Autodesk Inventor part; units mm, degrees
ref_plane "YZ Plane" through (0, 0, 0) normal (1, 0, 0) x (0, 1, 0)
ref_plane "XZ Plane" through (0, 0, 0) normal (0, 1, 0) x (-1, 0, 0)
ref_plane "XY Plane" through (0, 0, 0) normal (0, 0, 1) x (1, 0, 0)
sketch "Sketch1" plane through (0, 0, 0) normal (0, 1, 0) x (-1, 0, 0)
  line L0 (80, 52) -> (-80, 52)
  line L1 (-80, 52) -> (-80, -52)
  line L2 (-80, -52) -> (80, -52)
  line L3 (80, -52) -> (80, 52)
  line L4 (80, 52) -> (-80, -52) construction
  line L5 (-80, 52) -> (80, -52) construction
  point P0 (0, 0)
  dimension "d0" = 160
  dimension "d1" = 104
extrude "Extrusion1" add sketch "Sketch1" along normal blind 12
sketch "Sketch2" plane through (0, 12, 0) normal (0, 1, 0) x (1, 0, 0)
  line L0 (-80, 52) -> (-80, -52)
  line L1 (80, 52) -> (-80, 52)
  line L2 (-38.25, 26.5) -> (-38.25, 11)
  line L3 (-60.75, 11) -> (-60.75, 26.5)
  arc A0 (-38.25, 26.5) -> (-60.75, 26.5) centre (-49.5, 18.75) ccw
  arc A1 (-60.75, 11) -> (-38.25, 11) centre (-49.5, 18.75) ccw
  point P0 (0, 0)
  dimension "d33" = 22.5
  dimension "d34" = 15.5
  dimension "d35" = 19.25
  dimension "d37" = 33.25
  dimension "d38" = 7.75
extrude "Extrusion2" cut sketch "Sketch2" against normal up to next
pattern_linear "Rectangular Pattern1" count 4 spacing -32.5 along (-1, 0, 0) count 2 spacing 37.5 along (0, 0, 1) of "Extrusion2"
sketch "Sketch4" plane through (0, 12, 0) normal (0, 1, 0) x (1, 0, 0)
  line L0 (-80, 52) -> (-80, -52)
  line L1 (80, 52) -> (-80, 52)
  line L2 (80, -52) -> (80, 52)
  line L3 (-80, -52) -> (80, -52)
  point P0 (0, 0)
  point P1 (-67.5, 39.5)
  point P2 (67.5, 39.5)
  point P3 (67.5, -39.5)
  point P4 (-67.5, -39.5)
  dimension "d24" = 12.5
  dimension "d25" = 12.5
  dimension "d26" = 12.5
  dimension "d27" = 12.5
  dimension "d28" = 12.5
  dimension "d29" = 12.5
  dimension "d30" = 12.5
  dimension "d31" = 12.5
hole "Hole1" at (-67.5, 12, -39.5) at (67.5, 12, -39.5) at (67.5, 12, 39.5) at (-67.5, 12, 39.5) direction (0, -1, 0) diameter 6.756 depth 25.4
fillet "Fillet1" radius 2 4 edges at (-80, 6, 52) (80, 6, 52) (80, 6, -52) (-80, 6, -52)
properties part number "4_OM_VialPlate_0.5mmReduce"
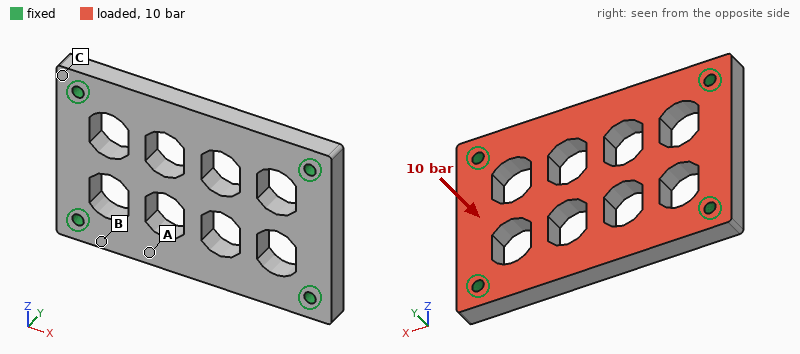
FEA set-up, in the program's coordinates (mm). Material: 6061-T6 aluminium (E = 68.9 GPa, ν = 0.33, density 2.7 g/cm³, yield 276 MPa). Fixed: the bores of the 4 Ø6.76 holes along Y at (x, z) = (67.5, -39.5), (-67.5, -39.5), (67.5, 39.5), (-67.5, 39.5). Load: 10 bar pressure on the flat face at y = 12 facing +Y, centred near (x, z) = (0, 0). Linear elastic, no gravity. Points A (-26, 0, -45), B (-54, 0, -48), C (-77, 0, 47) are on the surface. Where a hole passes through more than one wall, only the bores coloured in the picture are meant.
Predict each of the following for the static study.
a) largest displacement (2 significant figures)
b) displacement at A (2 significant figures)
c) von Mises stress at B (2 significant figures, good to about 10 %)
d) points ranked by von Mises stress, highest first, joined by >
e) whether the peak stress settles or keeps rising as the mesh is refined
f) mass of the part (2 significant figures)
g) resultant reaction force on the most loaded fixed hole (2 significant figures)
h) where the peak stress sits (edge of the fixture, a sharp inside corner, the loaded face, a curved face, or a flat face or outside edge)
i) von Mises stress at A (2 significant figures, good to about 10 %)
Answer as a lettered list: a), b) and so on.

a) 0.14 mm
b) 0.091 mm
c) 37 MPa
d) B > A > C
e) keeps rising
f) 400 g
g) 3.1 kN
h) edge of the fixture
i) 24 MPa
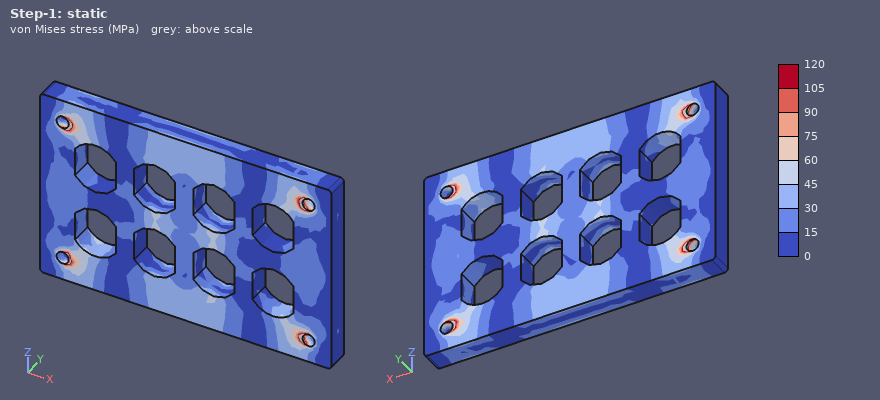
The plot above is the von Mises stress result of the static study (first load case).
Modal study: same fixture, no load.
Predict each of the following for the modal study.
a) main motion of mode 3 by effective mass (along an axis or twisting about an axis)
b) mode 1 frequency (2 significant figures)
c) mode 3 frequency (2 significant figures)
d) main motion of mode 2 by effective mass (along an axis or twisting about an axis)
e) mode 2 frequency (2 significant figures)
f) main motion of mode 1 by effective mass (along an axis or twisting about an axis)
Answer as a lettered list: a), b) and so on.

a) along Z
b) 2700 Hz
c) 6000 Hz
d) twisting about X
e) 3700 Hz
f) along Y
